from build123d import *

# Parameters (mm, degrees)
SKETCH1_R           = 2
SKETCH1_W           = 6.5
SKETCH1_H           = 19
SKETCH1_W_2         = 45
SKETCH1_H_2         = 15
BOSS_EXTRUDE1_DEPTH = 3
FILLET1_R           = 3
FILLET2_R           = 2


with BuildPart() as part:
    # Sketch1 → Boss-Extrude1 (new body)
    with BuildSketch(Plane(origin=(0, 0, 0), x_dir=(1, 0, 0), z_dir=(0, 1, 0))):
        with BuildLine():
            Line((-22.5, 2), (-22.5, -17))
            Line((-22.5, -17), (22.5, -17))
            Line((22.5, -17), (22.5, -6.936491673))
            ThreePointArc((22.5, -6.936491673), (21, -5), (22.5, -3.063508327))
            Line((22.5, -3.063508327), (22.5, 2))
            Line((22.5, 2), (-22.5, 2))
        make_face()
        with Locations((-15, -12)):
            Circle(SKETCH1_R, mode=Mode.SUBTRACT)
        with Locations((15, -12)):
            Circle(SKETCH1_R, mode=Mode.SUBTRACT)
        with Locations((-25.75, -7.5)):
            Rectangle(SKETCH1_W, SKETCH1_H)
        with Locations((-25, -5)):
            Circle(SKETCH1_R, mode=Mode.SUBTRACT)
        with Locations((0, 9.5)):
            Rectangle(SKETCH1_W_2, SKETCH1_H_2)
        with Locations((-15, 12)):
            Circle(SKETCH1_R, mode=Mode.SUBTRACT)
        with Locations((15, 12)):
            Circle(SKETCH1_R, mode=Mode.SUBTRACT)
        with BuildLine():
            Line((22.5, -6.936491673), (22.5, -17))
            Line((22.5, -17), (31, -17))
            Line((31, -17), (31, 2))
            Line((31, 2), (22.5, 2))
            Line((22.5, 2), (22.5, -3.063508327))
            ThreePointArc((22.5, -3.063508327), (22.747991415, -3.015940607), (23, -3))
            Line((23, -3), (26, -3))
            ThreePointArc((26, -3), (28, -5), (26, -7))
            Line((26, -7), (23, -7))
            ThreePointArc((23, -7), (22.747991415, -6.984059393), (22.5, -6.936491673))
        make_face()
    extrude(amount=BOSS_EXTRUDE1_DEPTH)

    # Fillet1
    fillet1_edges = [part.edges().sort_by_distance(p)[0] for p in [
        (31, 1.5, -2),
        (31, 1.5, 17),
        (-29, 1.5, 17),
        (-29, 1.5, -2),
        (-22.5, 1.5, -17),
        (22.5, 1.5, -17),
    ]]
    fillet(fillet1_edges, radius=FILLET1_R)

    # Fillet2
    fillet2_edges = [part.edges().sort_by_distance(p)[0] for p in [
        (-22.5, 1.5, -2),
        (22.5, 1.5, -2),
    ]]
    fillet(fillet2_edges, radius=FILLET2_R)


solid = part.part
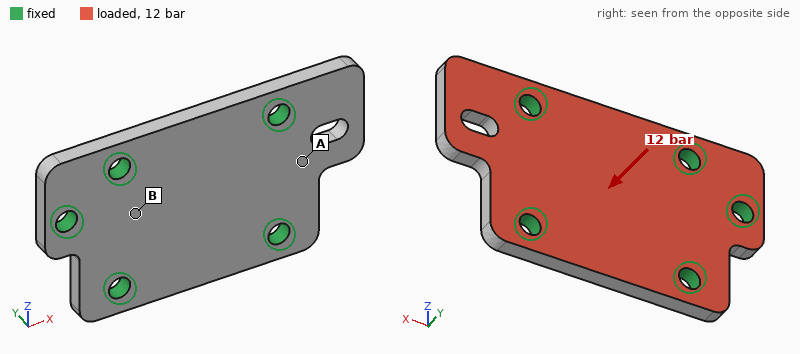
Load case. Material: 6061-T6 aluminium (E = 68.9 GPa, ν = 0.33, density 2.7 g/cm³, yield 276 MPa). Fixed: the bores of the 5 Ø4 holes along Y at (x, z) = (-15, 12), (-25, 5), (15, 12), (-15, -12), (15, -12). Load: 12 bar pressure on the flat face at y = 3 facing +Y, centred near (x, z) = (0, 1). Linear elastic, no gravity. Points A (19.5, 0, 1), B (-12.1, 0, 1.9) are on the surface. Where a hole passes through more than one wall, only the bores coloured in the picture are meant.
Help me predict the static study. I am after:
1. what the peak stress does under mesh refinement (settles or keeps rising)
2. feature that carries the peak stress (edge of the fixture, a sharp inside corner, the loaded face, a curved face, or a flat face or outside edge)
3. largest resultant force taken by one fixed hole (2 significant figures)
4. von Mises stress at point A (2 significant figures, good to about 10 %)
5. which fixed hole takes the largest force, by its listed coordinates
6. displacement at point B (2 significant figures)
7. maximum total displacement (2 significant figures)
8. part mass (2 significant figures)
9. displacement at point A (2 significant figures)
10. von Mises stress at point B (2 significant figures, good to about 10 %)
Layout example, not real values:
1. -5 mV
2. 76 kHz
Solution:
1. keeps rising
2. edge of the fixture
3. 590 N
4. 42 MPa
5. (15, 12)
6. 9.3 µm
7. 49 µm
8. 14 g
9. 14 µm
10. 17 MPa
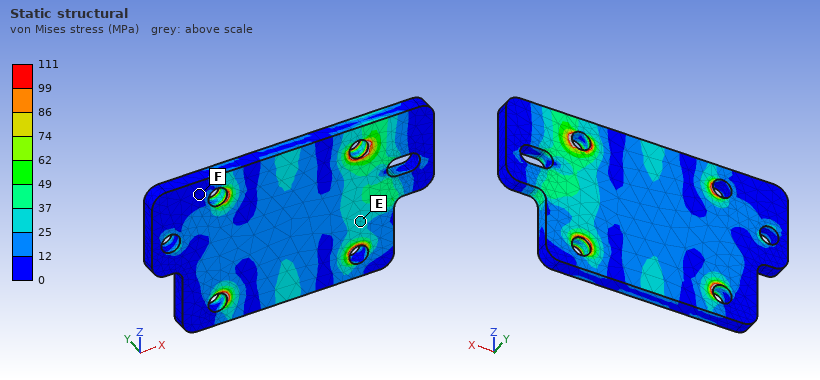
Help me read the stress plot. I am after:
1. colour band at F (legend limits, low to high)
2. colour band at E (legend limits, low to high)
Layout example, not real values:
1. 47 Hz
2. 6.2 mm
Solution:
1. 0 to 12 MPa
2. 25 to 37 MPa
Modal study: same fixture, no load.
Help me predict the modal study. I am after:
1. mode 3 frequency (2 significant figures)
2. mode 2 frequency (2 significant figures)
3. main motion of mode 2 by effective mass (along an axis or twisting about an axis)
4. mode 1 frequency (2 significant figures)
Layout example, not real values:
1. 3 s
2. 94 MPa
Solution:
1. 19 kHz
2. 16 kHz
3. along Y
4. 11 kHz
